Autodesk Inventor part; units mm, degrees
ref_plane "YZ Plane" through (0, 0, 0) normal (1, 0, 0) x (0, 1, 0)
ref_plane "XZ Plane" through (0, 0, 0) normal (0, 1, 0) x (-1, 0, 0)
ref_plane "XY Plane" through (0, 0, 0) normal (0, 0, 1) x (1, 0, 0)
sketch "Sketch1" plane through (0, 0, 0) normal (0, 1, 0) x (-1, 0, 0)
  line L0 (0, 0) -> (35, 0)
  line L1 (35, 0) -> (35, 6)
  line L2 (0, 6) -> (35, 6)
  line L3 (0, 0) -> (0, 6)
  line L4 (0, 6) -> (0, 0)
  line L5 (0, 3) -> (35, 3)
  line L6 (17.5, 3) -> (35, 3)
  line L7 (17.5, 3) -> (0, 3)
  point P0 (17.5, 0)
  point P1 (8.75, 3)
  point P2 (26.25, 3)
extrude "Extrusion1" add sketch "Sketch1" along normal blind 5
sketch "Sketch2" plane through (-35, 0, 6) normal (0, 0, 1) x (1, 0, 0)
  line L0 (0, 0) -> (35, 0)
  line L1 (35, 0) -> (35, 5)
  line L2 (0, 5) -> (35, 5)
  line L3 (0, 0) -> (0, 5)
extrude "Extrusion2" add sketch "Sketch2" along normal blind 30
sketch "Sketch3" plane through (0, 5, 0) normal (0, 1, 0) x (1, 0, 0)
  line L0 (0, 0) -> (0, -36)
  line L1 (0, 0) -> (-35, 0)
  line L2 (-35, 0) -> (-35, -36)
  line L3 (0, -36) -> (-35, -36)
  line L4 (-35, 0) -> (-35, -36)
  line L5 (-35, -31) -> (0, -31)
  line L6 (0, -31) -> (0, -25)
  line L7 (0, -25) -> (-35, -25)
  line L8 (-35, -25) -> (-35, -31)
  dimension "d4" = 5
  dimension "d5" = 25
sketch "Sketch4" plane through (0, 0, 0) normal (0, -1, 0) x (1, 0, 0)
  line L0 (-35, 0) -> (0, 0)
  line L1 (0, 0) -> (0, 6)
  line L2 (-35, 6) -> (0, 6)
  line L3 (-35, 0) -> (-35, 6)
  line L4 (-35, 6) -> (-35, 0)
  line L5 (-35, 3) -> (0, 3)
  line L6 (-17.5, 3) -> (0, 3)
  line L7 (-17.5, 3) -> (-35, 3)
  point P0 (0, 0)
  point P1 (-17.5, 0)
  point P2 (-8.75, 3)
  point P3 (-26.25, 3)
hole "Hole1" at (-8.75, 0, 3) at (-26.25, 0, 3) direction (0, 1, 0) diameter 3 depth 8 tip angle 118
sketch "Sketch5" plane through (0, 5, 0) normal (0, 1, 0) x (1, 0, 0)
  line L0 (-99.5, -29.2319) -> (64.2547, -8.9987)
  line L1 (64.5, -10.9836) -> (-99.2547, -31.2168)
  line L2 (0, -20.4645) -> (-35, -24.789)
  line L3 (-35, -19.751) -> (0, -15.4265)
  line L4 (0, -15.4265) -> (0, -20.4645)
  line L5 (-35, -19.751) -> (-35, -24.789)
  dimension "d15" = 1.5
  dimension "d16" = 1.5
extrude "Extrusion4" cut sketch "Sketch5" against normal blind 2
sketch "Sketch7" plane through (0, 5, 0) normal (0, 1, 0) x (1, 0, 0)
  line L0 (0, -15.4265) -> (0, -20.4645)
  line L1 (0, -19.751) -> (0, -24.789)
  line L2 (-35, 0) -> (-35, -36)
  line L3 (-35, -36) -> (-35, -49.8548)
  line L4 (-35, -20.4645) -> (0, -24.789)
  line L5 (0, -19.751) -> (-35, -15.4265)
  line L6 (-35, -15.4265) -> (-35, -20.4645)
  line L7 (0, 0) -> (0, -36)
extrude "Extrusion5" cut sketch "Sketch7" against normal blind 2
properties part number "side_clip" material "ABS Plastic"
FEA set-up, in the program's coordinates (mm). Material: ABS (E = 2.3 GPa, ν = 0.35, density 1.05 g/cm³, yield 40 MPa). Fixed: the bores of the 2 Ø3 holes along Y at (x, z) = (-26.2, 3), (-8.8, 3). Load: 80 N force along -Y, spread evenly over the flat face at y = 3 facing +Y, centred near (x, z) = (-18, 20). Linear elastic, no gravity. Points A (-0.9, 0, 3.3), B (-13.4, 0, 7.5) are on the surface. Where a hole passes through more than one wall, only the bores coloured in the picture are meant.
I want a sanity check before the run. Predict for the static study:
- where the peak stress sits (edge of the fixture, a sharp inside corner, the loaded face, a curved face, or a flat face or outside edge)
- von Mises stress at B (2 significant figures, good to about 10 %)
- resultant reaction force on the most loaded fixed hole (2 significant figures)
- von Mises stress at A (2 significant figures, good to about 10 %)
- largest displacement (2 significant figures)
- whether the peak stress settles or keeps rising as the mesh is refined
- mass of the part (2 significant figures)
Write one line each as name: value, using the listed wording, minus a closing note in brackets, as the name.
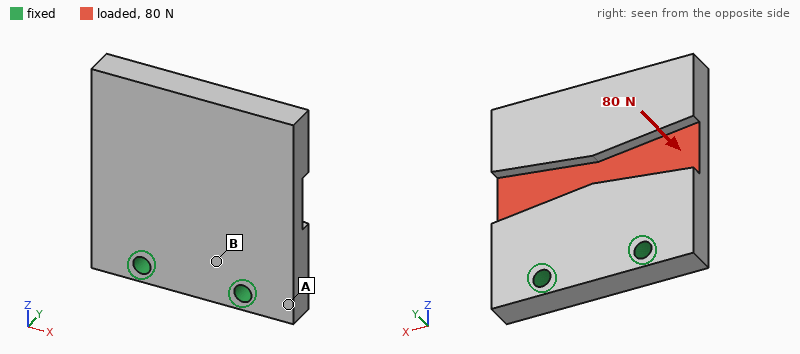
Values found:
where the peak stress sits: edge of the fixture
von Mises stress at B: 5.6 MPa
resultant reaction force on the most loaded fixed hole: 40 N
von Mises stress at A: 2.4 MPa
largest displacement: 0.54 mm
whether the peak stress settles or keeps rising as the mesh is refined: keeps rising
mass of the part: 6.0 g
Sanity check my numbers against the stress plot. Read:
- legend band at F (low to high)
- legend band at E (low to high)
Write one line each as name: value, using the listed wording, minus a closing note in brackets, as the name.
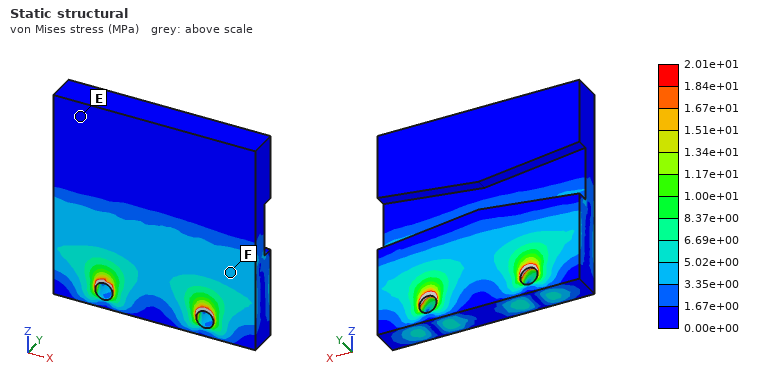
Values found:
legend band at F: 3.35e+00 to 5.02e+00 MPa
legend band at E: 0.00e+00 to 1.67e+00 MPa
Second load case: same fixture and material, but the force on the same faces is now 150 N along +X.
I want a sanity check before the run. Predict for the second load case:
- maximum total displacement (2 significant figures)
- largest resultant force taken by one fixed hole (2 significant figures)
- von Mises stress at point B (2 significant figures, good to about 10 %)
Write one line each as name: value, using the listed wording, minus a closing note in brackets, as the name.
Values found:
maximum total displacement: 93 µm
largest resultant force taken by one fixed hole: 150 N
von Mises stress at point B: 2.7 MPa
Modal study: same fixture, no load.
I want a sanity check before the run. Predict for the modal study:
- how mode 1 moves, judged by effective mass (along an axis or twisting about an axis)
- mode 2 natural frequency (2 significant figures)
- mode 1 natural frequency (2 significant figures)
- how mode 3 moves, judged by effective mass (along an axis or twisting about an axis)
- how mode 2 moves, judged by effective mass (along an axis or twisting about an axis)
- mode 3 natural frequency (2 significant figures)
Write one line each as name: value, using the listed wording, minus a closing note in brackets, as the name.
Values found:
how mode 1 moves, judged by effective mass: along Y
mode 2 natural frequency: 2000 Hz
mode 1 natural frequency: 880 Hz
how mode 3 moves, judged by effective mass: along X
how mode 2 moves, judged by effective mass: twisting about Z
mode 3 natural frequency: 3500 Hz
